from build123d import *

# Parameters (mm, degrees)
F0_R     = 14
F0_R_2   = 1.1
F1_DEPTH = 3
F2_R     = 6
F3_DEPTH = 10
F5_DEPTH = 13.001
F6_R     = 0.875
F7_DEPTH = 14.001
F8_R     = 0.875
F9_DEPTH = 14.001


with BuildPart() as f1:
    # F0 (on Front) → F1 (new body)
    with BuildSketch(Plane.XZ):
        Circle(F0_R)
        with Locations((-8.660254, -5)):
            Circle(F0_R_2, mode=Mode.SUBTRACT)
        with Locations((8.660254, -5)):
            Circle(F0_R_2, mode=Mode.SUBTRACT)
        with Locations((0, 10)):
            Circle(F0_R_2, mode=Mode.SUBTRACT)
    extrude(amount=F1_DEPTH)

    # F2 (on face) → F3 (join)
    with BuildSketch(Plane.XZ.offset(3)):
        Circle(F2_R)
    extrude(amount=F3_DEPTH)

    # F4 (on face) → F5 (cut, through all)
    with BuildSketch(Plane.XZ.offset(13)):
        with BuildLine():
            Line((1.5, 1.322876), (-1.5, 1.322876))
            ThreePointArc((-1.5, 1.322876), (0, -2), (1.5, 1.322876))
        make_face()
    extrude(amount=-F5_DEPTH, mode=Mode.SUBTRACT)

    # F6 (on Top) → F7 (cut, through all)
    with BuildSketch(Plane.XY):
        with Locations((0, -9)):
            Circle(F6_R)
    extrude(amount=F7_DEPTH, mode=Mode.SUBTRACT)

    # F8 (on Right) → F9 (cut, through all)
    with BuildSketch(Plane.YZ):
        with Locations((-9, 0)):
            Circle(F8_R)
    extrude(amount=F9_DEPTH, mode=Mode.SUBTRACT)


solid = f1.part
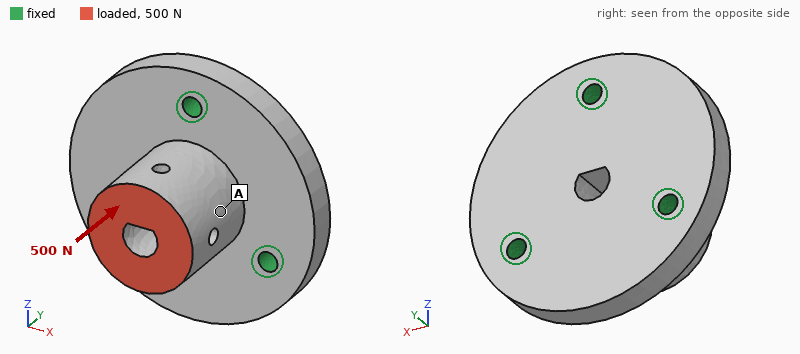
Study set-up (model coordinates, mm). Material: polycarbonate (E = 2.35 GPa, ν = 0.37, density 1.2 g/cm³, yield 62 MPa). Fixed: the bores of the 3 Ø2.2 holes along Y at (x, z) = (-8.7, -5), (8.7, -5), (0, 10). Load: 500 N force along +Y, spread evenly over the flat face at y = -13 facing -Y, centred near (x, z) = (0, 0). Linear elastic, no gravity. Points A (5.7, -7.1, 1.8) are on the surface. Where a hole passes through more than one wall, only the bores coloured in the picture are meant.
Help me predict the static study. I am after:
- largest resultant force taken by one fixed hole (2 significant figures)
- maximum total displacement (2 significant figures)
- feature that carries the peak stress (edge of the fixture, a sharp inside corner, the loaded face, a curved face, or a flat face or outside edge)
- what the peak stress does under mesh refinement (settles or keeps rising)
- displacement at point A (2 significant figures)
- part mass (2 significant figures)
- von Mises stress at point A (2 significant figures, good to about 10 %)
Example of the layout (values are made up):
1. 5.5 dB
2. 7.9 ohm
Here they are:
1. 170 N
2. 0.11 mm
3. edge of the fixture
4. keeps rising
5. 0.093 mm
6. 3.3 g
7. 5.9 MPa
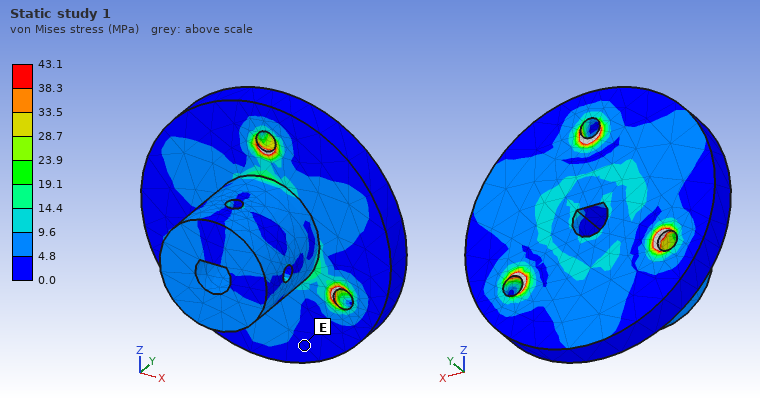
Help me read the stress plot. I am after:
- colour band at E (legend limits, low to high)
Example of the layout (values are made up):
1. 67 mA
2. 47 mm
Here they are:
1. 0.0 to 4.8 MPa
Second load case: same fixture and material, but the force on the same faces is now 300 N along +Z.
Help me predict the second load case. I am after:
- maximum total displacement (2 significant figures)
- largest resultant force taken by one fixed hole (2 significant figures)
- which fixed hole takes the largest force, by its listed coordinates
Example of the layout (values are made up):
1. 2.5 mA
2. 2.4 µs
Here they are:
1. 0.32 mm
2. 270 N
3. (0, 10)
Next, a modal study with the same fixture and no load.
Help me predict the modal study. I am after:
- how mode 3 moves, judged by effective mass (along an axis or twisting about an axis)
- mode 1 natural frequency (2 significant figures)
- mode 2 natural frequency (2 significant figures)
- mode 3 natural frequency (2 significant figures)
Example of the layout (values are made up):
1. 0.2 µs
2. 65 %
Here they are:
1. along Y
2. 6400 Hz
3. 6400 Hz
4. 7800 Hz
